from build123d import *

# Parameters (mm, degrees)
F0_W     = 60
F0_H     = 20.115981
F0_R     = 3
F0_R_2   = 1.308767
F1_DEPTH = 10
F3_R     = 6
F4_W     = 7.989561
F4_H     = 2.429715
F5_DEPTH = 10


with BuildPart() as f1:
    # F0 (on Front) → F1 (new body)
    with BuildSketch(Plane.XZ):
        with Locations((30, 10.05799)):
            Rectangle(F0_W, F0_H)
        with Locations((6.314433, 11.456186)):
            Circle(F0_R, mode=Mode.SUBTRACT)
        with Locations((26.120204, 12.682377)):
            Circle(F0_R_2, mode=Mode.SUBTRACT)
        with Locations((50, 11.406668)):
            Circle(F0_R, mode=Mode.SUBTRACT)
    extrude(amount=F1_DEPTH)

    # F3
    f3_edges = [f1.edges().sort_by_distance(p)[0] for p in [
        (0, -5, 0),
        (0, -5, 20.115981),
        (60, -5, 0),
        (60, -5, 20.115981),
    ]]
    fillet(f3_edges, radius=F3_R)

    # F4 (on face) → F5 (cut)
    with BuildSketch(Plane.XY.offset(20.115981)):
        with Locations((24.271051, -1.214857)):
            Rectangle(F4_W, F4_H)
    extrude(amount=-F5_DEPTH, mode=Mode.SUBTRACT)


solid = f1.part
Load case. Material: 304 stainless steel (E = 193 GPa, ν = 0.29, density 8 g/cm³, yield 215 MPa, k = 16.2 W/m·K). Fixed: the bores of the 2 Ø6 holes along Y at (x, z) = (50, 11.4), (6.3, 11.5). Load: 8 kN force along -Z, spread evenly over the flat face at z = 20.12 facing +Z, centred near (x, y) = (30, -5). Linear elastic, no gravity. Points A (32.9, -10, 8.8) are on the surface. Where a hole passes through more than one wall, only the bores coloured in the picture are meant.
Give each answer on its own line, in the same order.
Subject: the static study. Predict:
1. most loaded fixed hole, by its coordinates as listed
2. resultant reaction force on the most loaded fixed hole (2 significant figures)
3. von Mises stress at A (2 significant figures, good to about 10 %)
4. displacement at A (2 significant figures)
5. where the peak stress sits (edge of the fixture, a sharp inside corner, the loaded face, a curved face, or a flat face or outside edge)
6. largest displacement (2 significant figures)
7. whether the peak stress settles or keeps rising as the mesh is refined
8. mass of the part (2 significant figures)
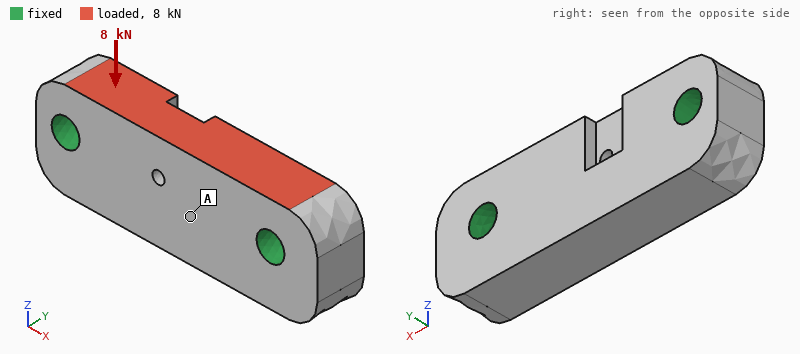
(50, 11.4)
4.4 kN
16 MPa
4.9 µm
edge of the fixture
6.0 µm
keeps rising
88 g
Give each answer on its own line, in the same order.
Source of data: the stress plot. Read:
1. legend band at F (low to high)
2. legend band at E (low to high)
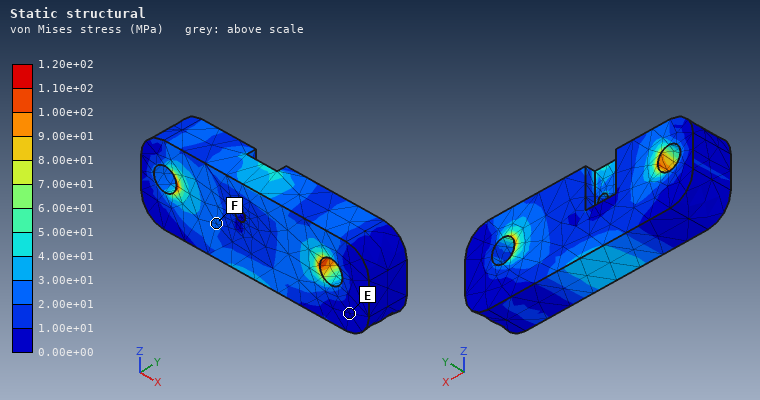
2.00e+01 to 3.00e+01 MPa
0.00e+00 to 1.00e+01 MPa
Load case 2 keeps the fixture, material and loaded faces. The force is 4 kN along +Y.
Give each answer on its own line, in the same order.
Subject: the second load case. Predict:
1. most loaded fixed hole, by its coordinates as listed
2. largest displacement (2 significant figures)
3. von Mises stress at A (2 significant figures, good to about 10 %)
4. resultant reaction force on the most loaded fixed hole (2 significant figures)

(50, 11.4)
11 µm
24 MPa
2.2 kN
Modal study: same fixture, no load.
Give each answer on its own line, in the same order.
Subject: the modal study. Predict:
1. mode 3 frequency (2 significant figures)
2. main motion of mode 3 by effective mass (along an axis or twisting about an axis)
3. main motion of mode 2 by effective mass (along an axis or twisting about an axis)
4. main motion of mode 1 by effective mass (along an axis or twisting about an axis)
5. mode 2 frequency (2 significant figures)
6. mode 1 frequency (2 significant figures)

27 kHz
twisting about X
along Z
along Y
25 kHz
20 kHz
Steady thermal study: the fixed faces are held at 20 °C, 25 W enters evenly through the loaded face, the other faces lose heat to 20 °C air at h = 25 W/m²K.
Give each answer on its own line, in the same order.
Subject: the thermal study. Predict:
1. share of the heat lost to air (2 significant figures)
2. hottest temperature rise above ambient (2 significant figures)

5.8 %
57 K
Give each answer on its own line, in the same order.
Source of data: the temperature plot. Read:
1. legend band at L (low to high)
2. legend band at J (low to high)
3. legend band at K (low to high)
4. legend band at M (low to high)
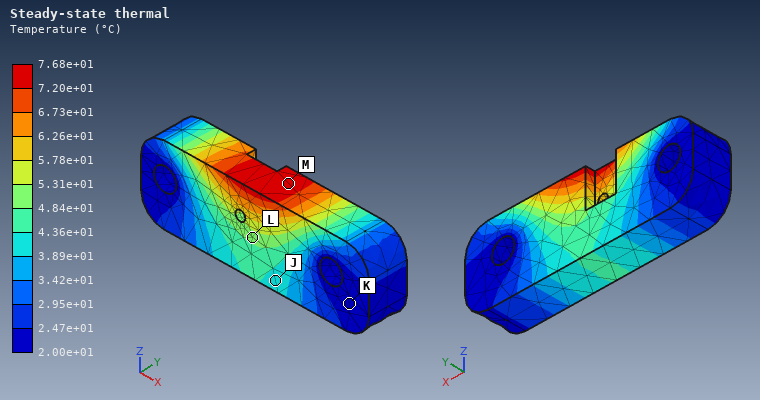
4.84e+01 to 5.31e+01 °C
3.89e+01 to 4.36e+01 °C
2.00e+01 to 2.47e+01 °C
7.20e+01 to 7.68e+01 °C
